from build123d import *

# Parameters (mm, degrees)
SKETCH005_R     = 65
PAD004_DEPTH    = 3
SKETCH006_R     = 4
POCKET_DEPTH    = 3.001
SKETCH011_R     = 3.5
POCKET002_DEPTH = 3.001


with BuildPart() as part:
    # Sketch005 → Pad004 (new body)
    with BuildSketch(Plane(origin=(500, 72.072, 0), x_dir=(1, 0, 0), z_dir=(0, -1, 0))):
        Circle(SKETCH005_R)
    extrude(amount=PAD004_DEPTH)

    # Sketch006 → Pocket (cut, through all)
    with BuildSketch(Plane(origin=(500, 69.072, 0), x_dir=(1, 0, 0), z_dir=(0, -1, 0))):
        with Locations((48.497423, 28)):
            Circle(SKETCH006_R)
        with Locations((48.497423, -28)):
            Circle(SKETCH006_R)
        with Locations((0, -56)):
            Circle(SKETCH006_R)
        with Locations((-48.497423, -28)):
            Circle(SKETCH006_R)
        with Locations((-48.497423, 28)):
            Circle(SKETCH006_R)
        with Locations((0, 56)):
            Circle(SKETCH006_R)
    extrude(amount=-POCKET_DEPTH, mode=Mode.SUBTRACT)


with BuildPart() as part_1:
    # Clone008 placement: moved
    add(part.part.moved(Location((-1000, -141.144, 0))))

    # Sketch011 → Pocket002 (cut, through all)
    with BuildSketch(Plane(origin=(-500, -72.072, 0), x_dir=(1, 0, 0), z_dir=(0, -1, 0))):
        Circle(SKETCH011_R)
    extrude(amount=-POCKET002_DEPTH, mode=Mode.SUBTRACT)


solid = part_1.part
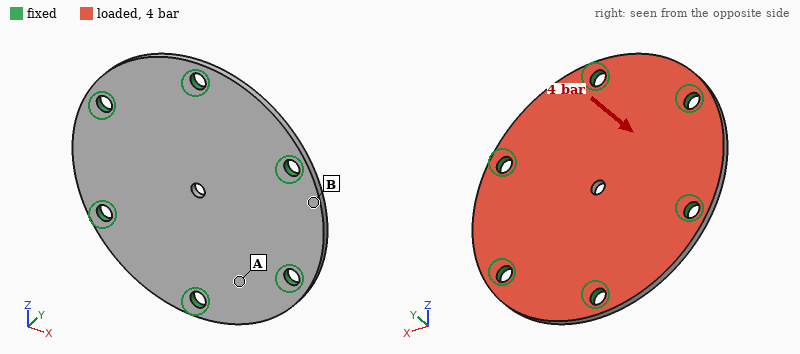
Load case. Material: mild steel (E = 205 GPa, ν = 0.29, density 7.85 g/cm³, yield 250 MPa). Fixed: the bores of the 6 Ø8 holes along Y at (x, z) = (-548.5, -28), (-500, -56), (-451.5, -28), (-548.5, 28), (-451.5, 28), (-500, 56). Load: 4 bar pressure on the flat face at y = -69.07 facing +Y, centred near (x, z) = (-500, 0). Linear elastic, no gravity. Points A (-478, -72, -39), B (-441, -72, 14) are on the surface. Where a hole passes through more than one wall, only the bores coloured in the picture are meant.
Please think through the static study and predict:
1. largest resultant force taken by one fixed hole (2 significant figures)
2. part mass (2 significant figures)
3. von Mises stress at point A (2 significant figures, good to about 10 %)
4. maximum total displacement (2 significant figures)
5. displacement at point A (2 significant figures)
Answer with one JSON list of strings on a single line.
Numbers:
["860 N", "300 g", "57 MPa", "0.14 mm", "0.033 mm"]
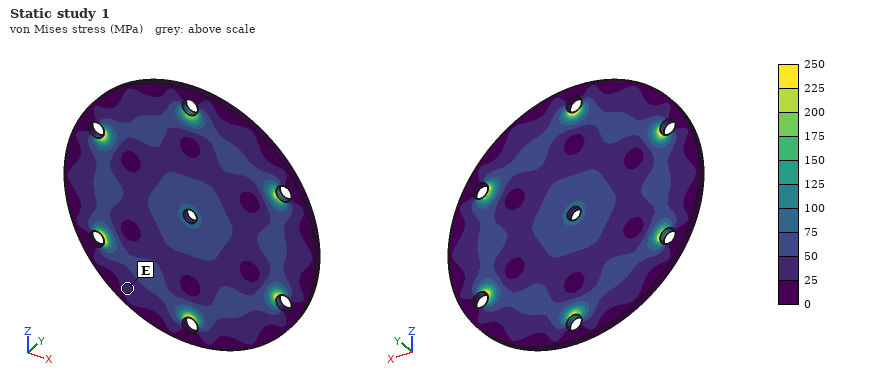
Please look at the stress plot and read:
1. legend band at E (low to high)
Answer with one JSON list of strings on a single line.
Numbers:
["25 to 50 MPa"]
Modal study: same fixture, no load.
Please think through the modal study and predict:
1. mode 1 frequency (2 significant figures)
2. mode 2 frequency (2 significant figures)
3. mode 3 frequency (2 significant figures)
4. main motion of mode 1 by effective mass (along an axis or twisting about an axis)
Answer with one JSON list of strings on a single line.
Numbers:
["2200 Hz", "4500 Hz", "4500 Hz", "along Y"]
